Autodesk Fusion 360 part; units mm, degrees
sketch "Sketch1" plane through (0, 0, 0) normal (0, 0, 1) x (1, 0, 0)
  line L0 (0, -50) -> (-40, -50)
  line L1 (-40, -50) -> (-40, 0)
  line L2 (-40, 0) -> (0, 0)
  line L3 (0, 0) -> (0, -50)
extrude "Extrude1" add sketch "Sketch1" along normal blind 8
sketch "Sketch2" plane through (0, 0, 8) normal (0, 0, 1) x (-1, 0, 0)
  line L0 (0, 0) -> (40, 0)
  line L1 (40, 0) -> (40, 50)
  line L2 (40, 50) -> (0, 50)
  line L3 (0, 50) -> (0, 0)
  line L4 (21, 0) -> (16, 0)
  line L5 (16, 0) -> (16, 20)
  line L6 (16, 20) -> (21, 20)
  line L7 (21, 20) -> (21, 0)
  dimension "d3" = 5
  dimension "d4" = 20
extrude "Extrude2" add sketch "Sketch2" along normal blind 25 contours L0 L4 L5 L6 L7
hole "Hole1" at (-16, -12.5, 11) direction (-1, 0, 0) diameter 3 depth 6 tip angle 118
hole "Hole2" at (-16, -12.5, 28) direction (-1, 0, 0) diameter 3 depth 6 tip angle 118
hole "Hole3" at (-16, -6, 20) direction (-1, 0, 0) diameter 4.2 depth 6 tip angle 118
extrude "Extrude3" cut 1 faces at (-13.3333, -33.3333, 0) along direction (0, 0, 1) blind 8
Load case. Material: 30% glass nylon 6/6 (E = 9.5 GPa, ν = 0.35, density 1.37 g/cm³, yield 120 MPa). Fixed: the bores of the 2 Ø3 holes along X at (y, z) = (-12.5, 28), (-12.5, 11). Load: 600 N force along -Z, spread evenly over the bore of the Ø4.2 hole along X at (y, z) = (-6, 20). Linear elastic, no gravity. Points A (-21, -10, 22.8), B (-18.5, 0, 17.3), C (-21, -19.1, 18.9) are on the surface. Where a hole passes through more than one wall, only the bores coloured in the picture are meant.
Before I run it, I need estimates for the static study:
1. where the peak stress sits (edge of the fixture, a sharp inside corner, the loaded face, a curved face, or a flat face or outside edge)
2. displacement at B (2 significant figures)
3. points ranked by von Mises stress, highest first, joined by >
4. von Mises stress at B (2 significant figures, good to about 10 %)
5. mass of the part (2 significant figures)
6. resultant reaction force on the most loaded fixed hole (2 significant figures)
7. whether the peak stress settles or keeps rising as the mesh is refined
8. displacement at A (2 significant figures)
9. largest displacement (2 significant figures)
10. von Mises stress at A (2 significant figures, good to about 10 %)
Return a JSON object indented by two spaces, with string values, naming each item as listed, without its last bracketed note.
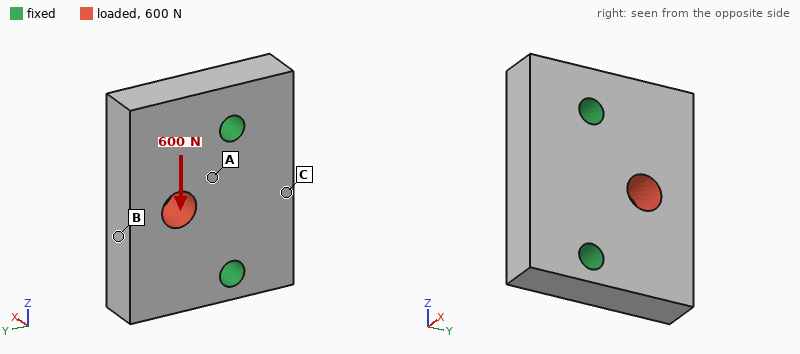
{
  "where the peak stress sits": "edge of the fixture",
  "displacement at B": "15 µm",
  "points ranked by von Mises stress, highest first, joined by >": "A > B > C",
  "von Mises stress at B": "4.7 MPa",
  "mass of the part": "3.2 g",
  "resultant reaction force on the most loaded fixed hole": "380 N",
  "whether the peak stress settles or keeps rising as the mesh is refined": "keeps rising",
  "displacement at A": "5.0 µm",
  "largest displacement": "18 µm",
  "von Mises stress at A": "9.5 MPa"
}
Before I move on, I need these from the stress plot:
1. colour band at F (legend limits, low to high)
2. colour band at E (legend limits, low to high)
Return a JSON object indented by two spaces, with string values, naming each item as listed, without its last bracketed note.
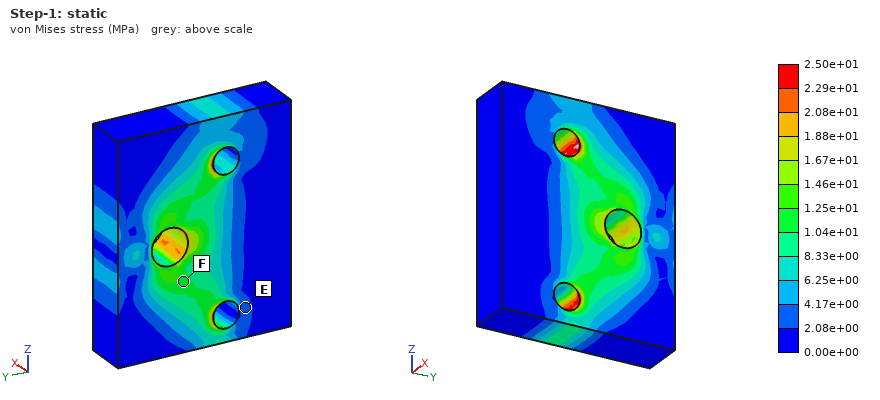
{
  "colour band at F": "1.04e+01 to 1.25e+01 MPa",
  "colour band at E": "2.08e+00 to 4.17e+00 MPa"
}
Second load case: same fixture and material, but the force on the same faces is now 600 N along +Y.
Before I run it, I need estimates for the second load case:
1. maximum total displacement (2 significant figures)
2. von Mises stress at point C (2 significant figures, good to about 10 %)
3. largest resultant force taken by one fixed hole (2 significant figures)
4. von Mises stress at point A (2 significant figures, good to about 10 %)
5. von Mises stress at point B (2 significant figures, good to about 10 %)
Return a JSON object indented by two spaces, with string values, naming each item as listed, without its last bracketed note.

{
  "maximum total displacement": "15 µm",
  "von Mises stress at point C": "4.2 MPa",
  "largest resultant force taken by one fixed hole": "330 N",
  "von Mises stress at point A": "7.7 MPa",
  "von Mises stress at point B": "8.0 MPa"
}
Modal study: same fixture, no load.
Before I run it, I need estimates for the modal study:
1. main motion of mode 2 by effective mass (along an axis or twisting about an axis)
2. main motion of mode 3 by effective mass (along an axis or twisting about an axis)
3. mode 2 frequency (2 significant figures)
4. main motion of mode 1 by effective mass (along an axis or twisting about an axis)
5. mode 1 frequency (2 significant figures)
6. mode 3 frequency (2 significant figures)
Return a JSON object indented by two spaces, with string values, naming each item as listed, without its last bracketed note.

{
  "main motion of mode 2 by effective mass": "twisting about Y",
  "main motion of mode 3 by effective mass": "along Z",
  "mode 2 frequency": "17 kHz",
  "main motion of mode 1 by effective mass": "along X",
  "mode 1 frequency": "11 kHz",
  "mode 3 frequency": "24 kHz"
}
